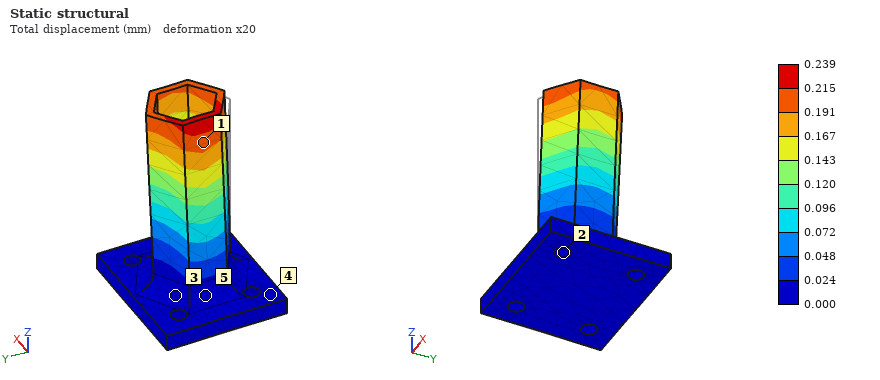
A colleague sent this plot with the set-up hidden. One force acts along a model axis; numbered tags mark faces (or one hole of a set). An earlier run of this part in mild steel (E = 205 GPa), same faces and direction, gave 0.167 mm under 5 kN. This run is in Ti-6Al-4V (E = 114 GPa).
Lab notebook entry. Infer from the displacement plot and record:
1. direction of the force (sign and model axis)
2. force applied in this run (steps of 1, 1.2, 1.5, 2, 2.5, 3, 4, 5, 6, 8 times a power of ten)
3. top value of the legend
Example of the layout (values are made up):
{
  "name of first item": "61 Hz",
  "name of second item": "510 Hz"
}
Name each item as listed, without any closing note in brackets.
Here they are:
{
  "direction of the force": "+X",
  "force applied in this run": "4 kN",
  "top value of the legend": "0.239 mm"
}
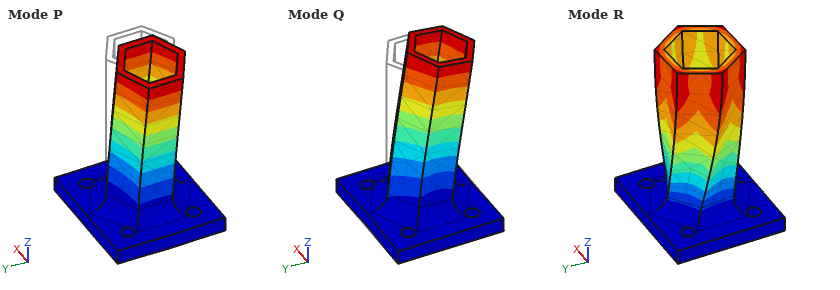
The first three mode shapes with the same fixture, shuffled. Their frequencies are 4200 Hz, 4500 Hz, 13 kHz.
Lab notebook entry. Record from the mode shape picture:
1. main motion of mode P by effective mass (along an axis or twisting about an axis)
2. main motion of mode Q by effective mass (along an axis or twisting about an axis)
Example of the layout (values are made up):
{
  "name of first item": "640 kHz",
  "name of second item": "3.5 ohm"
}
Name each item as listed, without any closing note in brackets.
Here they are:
{
  "main motion of mode P by effective mass": "along X",
  "main motion of mode Q by effective mass": "along Y"
}
